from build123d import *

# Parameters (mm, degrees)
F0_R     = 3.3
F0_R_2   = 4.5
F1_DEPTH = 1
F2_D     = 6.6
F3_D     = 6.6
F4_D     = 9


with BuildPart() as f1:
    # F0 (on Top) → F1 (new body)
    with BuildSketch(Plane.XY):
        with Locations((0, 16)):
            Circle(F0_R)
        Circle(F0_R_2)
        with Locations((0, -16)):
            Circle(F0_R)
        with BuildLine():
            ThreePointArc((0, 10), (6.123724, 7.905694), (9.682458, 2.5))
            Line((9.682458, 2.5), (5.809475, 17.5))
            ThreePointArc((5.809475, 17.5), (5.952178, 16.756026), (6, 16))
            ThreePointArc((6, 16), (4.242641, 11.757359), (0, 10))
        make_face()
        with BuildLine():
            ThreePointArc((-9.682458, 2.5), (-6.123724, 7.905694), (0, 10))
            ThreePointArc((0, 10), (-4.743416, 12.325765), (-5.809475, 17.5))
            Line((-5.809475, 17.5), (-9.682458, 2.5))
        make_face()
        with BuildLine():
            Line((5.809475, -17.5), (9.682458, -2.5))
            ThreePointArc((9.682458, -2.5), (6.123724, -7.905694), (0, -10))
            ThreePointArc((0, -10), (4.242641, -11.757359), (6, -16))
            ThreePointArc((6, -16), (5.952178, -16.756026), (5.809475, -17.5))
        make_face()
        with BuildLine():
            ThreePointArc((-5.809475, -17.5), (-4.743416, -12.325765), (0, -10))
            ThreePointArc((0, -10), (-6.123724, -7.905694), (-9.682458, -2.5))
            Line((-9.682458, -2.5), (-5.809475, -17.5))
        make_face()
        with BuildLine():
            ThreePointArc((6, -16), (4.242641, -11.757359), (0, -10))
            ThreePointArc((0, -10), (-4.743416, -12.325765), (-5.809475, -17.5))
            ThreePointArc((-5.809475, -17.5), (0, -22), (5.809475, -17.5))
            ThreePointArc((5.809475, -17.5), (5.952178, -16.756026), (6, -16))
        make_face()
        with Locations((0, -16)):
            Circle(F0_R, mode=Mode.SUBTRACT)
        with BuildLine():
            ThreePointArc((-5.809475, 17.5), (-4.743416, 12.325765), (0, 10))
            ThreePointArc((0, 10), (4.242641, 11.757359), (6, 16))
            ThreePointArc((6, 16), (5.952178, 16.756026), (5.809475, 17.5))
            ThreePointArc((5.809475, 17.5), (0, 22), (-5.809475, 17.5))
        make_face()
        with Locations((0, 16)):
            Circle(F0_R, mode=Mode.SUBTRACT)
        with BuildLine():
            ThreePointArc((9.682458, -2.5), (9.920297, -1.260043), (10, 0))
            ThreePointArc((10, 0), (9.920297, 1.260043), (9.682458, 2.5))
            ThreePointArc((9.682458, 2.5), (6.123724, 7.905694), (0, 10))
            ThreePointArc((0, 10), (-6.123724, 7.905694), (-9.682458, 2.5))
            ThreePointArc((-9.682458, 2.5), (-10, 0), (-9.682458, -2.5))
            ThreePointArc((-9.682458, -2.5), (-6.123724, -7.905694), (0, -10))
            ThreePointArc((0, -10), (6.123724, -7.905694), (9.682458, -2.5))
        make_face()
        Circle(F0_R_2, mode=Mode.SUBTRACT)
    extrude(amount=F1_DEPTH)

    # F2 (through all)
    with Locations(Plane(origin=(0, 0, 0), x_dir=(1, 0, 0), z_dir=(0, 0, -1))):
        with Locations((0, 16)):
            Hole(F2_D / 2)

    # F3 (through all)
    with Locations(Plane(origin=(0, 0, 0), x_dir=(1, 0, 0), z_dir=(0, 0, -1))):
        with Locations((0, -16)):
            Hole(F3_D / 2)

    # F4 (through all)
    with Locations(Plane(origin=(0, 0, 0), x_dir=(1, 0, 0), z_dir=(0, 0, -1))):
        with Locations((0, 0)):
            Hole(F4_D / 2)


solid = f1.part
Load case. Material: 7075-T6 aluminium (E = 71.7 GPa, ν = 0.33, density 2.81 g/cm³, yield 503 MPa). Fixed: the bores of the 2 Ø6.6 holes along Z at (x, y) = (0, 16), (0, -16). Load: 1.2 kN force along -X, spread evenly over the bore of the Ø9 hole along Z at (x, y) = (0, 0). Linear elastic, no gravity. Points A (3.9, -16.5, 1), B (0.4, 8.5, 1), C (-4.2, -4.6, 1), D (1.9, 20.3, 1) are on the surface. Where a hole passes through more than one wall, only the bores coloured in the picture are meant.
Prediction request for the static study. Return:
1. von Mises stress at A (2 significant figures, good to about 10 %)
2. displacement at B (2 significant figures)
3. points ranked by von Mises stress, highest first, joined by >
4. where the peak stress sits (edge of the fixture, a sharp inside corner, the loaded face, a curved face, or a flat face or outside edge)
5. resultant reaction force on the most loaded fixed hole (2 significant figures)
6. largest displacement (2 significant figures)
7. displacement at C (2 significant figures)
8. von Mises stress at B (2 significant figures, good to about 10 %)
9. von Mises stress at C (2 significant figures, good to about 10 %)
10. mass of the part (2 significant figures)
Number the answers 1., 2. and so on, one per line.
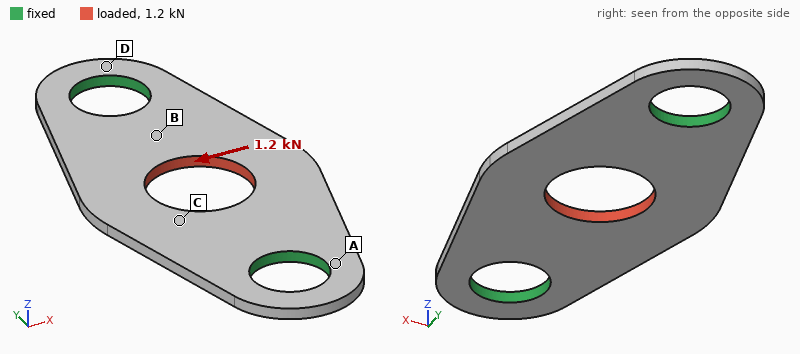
1. 39 MPa
2. 13 µm
3. B > C > A > D
4. edge of the fixture
5. 600 N
6. 26 µm
7. 21 µm
8. 86 MPa
9. 61 MPa
10. 1.4 g
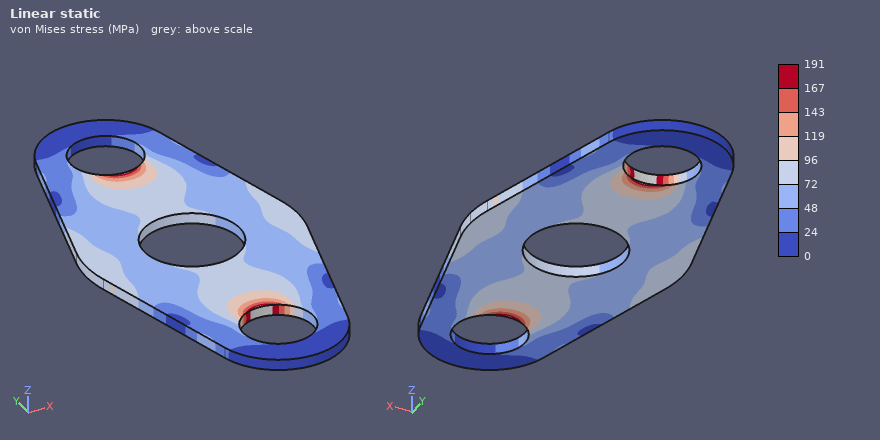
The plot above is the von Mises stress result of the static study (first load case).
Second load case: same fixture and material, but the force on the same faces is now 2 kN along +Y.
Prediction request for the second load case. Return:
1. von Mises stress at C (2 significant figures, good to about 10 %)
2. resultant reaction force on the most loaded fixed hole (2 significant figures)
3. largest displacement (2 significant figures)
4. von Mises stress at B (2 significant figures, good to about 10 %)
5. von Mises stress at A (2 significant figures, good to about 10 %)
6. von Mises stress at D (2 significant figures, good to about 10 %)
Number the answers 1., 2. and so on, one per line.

1. 84 MPa
2. 1.0 kN
3. 15 µm
4. 95 MPa
5. 46 MPa
6. 11 MPa
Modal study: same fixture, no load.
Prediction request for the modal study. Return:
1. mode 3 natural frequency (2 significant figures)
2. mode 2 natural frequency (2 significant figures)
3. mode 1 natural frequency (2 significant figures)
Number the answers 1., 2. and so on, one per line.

1. 16 kHz
2. 6700 Hz
3. 6400 Hz
